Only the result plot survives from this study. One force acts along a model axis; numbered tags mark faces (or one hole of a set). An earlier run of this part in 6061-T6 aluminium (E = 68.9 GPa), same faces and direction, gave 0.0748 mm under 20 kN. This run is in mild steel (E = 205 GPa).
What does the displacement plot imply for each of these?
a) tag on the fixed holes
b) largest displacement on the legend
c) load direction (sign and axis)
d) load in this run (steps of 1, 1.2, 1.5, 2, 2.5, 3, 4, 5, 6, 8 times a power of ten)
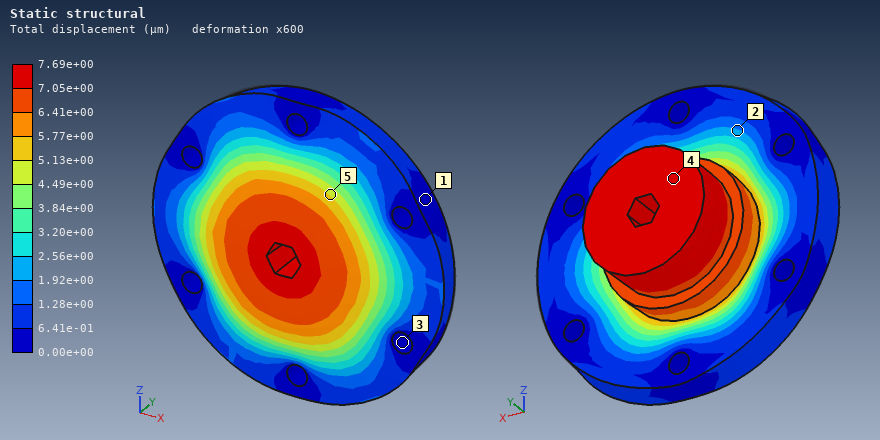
3
7.69e+00 µm
-Y
6 kN
